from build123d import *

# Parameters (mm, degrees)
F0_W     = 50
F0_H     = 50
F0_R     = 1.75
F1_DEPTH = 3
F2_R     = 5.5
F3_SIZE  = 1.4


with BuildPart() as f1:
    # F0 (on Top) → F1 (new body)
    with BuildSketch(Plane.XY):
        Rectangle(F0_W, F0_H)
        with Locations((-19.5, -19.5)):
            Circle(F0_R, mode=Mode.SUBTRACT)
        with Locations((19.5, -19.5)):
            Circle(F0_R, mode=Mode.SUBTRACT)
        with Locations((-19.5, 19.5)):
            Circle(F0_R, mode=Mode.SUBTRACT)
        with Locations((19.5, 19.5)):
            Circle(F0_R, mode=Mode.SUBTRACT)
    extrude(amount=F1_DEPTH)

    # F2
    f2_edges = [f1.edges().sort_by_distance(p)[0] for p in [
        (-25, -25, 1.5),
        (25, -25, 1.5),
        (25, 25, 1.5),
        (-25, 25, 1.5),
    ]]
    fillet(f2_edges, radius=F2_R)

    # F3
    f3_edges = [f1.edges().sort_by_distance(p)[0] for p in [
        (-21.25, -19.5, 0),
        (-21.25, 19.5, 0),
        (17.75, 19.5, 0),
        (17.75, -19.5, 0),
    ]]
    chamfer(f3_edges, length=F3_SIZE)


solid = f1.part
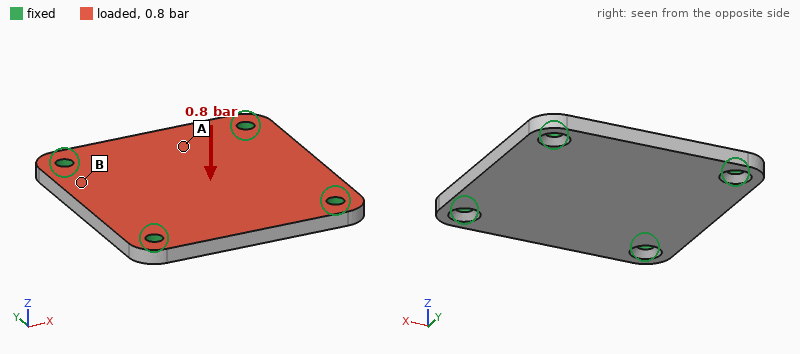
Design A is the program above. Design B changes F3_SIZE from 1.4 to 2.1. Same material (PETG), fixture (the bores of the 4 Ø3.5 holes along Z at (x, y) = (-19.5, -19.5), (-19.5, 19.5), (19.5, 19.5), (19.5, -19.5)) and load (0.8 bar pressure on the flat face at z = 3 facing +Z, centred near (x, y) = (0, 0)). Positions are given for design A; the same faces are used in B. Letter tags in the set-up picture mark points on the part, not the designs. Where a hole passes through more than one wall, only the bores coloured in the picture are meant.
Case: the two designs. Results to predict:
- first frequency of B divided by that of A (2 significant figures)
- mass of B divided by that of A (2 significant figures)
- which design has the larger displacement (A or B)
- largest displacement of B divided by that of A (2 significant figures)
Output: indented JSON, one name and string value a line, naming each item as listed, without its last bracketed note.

{
  "first frequency of B divided by that of A": "0.93",
  "mass of B divided by that of A": "0.99",
  "which design has the larger displacement": "B",
  "largest displacement of B divided by that of A": "1.1"
}
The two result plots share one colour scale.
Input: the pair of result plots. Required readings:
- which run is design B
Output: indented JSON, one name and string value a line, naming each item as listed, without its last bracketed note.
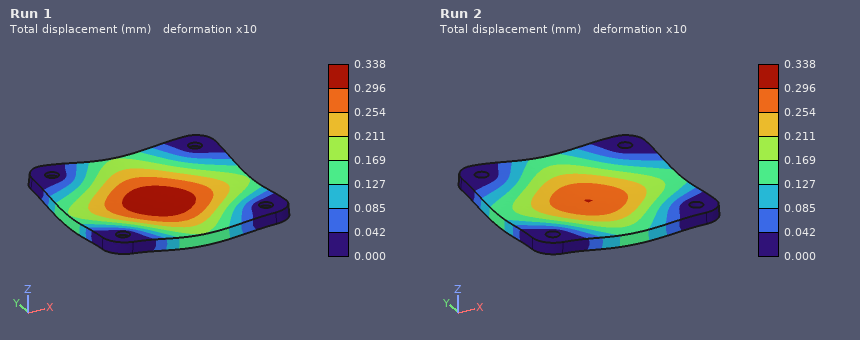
{
  "which run is design B": "Run 1"
}
